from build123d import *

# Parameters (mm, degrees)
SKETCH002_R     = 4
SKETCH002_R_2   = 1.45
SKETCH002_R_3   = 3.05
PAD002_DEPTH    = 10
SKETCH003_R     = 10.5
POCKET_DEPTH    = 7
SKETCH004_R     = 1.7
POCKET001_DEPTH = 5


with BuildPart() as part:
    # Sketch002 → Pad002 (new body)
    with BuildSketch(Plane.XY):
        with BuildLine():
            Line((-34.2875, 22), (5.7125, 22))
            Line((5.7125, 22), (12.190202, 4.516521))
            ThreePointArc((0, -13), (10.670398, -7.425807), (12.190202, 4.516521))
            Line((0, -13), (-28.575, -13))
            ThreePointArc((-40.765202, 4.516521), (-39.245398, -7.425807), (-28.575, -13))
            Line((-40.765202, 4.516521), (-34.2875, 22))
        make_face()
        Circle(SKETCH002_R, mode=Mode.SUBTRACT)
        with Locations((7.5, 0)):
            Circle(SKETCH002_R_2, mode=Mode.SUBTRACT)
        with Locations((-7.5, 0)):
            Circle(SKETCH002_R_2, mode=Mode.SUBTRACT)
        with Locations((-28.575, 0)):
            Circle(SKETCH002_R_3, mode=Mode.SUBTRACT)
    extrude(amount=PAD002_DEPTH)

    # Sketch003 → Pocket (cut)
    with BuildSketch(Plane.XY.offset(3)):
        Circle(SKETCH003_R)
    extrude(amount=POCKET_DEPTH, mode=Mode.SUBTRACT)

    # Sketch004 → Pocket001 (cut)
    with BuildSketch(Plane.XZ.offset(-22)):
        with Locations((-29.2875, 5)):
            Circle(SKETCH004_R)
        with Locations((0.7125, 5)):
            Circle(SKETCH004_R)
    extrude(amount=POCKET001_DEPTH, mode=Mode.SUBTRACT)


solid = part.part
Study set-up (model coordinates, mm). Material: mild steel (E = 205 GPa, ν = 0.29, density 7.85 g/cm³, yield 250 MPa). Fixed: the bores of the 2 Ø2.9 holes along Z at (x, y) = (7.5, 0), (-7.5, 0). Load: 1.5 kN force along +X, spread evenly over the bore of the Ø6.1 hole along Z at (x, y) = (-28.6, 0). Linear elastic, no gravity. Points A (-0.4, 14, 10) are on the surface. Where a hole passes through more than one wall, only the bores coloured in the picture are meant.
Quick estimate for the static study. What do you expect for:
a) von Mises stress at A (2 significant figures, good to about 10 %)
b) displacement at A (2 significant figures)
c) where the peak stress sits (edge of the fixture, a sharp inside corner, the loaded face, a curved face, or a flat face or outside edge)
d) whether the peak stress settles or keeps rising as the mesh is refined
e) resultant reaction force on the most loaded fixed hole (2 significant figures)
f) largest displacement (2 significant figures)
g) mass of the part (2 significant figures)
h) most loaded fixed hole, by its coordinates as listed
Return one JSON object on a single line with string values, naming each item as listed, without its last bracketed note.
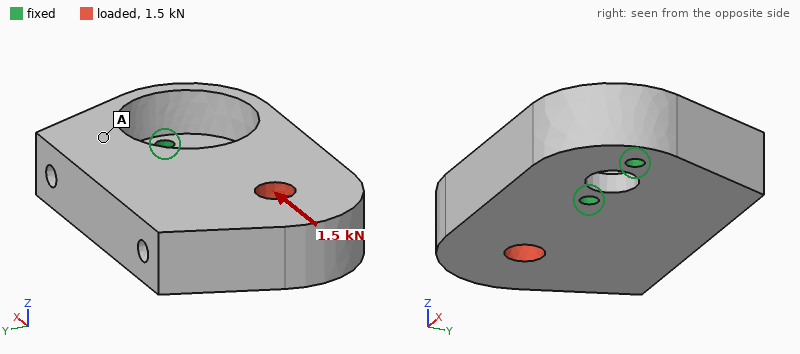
{"von Mises stress at A": "11 MPa", "displacement at A": "2.9 µm", "where the peak stress sits": "edge of the fixture", "whether the peak stress settles or keeps rising as the mesh is refined": "keeps rising", "resultant reaction force on the most loaded fixed hole": "1.1 kN", "largest displacement": "12 µm", "mass of the part": "110 g", "most loaded fixed hole, by its coordinates as listed": "(-7.5, 0)"}
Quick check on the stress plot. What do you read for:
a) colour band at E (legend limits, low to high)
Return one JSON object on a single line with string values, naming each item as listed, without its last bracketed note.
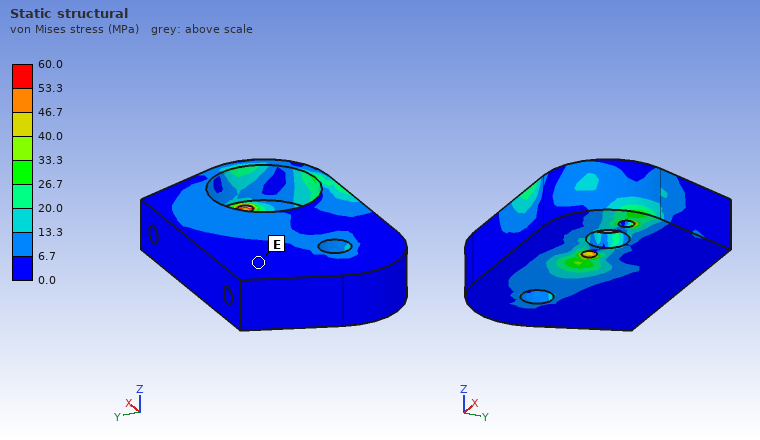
{"colour band at E": "0.0 to 6.7 MPa"}
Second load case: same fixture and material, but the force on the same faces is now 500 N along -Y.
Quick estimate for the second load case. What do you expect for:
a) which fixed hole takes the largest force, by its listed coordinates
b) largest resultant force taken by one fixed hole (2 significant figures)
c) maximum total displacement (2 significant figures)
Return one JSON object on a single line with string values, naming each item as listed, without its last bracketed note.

{"which fixed hole takes the largest force, by its listed coordinates": "(-7.5, 0)", "largest resultant force taken by one fixed hole": "1.1 kN", "maximum total displacement": "11 µm"}
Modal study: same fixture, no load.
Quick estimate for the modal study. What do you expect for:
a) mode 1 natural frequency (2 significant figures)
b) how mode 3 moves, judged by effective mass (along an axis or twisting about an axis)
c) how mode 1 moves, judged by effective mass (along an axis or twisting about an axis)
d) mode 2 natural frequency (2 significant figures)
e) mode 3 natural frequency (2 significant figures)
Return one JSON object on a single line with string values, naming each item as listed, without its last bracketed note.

{"mode 1 natural frequency": "2900 Hz", "how mode 3 moves, judged by effective mass": "along Y", "how mode 1 moves, judged by effective mass": "along Z", "mode 2 natural frequency": "3700 Hz", "mode 3 natural frequency": "6100 Hz"}
